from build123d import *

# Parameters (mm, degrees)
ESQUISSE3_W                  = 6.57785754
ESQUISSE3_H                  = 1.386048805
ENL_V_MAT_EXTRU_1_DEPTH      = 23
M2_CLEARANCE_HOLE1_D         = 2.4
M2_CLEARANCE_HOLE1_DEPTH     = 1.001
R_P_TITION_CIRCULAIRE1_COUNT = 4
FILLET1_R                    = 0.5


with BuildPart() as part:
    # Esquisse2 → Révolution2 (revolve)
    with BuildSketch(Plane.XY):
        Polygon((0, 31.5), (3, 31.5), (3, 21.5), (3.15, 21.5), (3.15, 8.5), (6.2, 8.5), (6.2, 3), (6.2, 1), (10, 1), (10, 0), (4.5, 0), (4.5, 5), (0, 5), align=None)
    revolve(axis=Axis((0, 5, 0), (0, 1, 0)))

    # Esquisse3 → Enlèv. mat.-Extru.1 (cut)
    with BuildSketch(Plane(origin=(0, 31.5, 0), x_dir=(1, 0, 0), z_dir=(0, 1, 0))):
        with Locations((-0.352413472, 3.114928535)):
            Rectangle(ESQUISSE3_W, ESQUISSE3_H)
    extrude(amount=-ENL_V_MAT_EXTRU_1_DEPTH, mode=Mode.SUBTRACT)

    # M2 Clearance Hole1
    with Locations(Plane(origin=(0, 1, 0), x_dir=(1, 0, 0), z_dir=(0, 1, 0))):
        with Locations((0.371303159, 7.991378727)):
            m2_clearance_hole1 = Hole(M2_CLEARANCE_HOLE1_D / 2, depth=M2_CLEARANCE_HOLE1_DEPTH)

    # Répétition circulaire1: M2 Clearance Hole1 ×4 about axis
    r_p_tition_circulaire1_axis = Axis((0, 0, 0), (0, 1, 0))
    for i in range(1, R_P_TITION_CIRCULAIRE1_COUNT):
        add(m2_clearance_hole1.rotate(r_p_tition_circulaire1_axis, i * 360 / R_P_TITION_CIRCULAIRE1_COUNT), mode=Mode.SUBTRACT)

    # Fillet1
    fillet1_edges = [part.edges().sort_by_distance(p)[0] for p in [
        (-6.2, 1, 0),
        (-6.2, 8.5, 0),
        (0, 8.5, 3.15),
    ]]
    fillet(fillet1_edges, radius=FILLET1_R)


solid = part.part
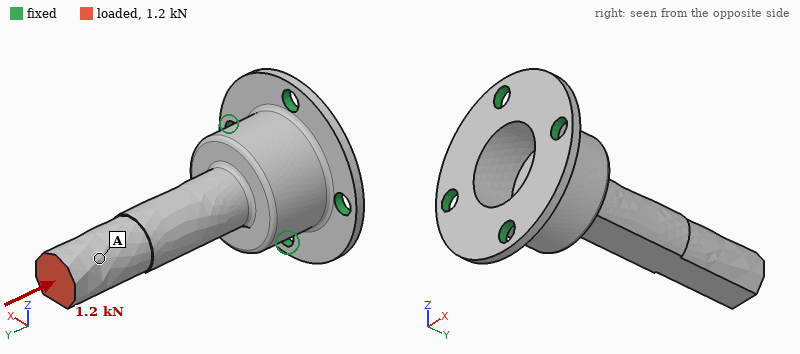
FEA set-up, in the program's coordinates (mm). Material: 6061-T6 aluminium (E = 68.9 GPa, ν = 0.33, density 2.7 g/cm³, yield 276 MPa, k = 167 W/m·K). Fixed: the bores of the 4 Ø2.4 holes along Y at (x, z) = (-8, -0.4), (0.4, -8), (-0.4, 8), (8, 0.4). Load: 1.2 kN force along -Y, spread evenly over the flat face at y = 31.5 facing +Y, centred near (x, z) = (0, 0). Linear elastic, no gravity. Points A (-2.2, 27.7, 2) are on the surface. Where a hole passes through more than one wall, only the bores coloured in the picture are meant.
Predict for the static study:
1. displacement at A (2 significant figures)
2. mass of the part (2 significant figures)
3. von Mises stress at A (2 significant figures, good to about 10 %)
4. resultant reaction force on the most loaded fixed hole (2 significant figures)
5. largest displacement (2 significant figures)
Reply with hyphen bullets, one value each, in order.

- 22 µm
- 4.1 g
- 44 MPa
- 340 N
- 26 µm
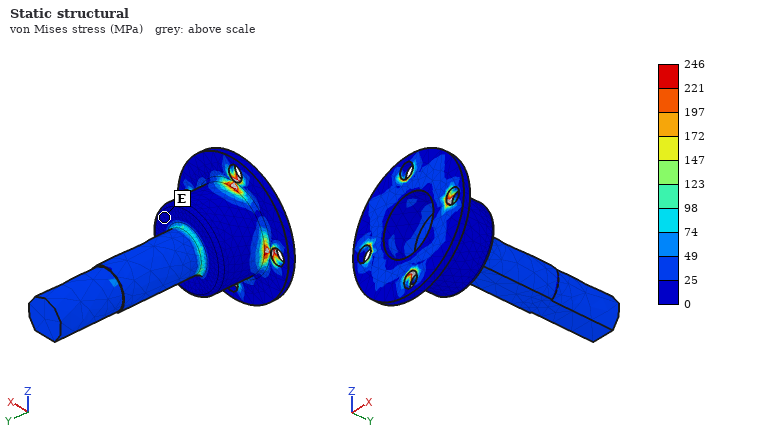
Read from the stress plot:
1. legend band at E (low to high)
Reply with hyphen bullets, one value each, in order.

- 0 to 25 MPa
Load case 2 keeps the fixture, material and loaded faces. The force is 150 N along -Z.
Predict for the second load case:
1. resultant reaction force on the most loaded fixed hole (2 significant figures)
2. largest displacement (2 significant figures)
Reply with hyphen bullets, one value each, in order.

- 360 N
- 0.23 mm
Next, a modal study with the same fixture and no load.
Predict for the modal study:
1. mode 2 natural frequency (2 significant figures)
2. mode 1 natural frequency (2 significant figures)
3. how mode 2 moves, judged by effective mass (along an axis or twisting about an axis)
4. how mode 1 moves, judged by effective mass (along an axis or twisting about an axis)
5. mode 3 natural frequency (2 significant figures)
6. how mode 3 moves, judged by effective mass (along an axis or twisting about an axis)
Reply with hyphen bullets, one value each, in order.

- 6200 Hz
- 5800 Hz
- along X
- along Z
- 24 kHz
- along Z
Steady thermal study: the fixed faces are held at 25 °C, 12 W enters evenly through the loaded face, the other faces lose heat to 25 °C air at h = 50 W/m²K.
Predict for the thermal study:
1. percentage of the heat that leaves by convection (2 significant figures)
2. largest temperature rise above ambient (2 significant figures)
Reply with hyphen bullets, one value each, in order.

- 10 %
- 70 K
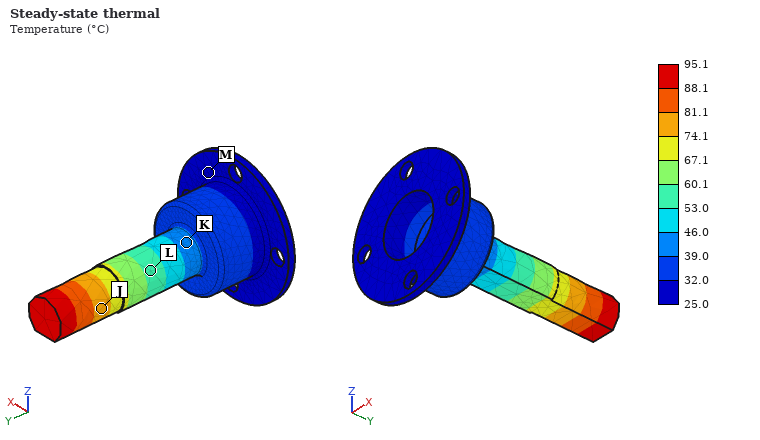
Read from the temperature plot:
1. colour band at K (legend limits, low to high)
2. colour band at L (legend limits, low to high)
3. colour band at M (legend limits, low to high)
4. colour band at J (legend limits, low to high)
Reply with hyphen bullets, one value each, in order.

- 39.0 to 46.0 °C
- 53.0 to 60.1 °C
- 25.0 to 32.0 °C
- 74.1 to 81.1 °C
